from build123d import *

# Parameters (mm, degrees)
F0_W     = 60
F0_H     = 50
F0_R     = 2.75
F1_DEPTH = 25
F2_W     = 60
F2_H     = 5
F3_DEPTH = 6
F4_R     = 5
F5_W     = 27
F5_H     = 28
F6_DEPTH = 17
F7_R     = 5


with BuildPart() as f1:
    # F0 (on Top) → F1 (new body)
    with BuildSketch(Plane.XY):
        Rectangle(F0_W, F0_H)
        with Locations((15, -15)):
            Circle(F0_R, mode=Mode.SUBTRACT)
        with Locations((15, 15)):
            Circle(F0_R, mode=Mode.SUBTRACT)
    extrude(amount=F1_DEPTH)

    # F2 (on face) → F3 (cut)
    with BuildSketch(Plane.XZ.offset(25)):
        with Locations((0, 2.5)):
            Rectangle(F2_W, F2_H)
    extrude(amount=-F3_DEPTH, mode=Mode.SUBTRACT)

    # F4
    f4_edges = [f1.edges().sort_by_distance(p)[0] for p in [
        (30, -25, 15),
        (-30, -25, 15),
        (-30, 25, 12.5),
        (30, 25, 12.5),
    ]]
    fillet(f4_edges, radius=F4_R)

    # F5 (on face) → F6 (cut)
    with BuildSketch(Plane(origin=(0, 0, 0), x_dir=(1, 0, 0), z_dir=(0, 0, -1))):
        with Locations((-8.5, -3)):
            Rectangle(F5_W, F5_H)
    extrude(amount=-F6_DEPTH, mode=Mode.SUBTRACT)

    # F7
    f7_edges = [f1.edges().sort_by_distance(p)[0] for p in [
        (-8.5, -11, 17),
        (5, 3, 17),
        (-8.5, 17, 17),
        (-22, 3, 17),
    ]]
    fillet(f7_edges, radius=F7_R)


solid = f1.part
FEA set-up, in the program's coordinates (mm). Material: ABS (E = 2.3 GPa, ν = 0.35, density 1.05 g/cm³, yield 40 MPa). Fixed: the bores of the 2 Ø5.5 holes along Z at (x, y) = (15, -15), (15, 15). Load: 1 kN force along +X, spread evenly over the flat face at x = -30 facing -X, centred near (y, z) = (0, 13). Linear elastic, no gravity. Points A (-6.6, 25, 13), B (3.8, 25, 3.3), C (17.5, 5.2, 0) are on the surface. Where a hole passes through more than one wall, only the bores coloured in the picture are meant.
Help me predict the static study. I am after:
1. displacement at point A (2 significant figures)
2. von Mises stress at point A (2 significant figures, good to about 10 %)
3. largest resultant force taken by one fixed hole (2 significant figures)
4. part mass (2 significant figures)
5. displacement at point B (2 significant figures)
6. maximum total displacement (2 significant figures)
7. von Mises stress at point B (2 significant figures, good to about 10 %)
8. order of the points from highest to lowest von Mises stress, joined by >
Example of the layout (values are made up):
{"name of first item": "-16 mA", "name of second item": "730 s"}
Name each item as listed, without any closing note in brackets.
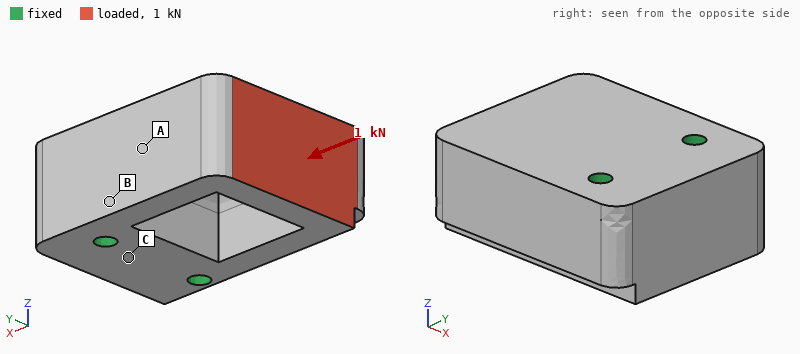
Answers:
{"displacement at point A": "0.022 mm", "von Mises stress at point A": "1.0 MPa", "largest resultant force taken by one fixed hole": "510 N", "part mass": "62 g", "displacement at point B": "0.021 mm", "maximum total displacement": "0.13 mm", "von Mises stress at point B": "2.3 MPa", "order of the points from highest to lowest von Mises stress, joined by >": "B > A > C"}
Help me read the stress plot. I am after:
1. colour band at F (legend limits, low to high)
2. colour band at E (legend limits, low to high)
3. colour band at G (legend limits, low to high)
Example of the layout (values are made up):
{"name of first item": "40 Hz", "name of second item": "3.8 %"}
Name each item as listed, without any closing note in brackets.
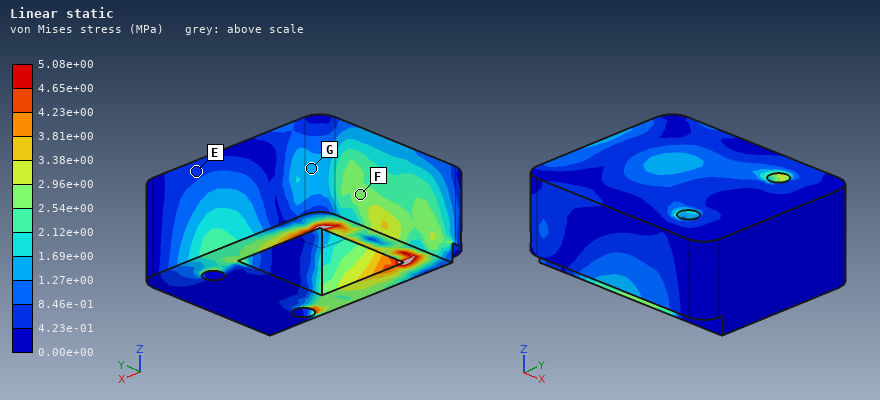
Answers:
{"colour band at F": "2.54e+00 to 2.96e+00 MPa", "colour band at E": "4.23e-01 to 8.46e-01 MPa", "colour band at G": "1.27e+00 to 1.69e+00 MPa"}
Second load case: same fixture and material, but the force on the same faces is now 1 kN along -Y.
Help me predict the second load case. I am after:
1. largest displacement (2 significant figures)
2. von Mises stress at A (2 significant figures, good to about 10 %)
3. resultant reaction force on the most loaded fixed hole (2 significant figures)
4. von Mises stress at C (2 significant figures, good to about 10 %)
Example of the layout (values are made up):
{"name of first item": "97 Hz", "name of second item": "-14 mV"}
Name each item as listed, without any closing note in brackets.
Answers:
{"largest displacement": "0.34 mm", "von Mises stress at A": "4.9 MPa", "resultant reaction force on the most loaded fixed hole": "1.4 kN", "von Mises stress at C": "1.4 MPa"}
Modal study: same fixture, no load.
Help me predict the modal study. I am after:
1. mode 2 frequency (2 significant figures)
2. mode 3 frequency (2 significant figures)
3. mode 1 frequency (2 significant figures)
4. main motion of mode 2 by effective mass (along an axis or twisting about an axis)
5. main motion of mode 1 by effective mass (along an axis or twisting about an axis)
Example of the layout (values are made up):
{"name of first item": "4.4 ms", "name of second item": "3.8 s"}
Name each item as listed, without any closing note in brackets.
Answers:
{"mode 2 frequency": "2400 Hz", "mode 3 frequency": "3700 Hz", "mode 1 frequency": "2000 Hz", "main motion of mode 2 by effective mass": "along Y", "main motion of mode 1 by effective mass": "along Z"}
